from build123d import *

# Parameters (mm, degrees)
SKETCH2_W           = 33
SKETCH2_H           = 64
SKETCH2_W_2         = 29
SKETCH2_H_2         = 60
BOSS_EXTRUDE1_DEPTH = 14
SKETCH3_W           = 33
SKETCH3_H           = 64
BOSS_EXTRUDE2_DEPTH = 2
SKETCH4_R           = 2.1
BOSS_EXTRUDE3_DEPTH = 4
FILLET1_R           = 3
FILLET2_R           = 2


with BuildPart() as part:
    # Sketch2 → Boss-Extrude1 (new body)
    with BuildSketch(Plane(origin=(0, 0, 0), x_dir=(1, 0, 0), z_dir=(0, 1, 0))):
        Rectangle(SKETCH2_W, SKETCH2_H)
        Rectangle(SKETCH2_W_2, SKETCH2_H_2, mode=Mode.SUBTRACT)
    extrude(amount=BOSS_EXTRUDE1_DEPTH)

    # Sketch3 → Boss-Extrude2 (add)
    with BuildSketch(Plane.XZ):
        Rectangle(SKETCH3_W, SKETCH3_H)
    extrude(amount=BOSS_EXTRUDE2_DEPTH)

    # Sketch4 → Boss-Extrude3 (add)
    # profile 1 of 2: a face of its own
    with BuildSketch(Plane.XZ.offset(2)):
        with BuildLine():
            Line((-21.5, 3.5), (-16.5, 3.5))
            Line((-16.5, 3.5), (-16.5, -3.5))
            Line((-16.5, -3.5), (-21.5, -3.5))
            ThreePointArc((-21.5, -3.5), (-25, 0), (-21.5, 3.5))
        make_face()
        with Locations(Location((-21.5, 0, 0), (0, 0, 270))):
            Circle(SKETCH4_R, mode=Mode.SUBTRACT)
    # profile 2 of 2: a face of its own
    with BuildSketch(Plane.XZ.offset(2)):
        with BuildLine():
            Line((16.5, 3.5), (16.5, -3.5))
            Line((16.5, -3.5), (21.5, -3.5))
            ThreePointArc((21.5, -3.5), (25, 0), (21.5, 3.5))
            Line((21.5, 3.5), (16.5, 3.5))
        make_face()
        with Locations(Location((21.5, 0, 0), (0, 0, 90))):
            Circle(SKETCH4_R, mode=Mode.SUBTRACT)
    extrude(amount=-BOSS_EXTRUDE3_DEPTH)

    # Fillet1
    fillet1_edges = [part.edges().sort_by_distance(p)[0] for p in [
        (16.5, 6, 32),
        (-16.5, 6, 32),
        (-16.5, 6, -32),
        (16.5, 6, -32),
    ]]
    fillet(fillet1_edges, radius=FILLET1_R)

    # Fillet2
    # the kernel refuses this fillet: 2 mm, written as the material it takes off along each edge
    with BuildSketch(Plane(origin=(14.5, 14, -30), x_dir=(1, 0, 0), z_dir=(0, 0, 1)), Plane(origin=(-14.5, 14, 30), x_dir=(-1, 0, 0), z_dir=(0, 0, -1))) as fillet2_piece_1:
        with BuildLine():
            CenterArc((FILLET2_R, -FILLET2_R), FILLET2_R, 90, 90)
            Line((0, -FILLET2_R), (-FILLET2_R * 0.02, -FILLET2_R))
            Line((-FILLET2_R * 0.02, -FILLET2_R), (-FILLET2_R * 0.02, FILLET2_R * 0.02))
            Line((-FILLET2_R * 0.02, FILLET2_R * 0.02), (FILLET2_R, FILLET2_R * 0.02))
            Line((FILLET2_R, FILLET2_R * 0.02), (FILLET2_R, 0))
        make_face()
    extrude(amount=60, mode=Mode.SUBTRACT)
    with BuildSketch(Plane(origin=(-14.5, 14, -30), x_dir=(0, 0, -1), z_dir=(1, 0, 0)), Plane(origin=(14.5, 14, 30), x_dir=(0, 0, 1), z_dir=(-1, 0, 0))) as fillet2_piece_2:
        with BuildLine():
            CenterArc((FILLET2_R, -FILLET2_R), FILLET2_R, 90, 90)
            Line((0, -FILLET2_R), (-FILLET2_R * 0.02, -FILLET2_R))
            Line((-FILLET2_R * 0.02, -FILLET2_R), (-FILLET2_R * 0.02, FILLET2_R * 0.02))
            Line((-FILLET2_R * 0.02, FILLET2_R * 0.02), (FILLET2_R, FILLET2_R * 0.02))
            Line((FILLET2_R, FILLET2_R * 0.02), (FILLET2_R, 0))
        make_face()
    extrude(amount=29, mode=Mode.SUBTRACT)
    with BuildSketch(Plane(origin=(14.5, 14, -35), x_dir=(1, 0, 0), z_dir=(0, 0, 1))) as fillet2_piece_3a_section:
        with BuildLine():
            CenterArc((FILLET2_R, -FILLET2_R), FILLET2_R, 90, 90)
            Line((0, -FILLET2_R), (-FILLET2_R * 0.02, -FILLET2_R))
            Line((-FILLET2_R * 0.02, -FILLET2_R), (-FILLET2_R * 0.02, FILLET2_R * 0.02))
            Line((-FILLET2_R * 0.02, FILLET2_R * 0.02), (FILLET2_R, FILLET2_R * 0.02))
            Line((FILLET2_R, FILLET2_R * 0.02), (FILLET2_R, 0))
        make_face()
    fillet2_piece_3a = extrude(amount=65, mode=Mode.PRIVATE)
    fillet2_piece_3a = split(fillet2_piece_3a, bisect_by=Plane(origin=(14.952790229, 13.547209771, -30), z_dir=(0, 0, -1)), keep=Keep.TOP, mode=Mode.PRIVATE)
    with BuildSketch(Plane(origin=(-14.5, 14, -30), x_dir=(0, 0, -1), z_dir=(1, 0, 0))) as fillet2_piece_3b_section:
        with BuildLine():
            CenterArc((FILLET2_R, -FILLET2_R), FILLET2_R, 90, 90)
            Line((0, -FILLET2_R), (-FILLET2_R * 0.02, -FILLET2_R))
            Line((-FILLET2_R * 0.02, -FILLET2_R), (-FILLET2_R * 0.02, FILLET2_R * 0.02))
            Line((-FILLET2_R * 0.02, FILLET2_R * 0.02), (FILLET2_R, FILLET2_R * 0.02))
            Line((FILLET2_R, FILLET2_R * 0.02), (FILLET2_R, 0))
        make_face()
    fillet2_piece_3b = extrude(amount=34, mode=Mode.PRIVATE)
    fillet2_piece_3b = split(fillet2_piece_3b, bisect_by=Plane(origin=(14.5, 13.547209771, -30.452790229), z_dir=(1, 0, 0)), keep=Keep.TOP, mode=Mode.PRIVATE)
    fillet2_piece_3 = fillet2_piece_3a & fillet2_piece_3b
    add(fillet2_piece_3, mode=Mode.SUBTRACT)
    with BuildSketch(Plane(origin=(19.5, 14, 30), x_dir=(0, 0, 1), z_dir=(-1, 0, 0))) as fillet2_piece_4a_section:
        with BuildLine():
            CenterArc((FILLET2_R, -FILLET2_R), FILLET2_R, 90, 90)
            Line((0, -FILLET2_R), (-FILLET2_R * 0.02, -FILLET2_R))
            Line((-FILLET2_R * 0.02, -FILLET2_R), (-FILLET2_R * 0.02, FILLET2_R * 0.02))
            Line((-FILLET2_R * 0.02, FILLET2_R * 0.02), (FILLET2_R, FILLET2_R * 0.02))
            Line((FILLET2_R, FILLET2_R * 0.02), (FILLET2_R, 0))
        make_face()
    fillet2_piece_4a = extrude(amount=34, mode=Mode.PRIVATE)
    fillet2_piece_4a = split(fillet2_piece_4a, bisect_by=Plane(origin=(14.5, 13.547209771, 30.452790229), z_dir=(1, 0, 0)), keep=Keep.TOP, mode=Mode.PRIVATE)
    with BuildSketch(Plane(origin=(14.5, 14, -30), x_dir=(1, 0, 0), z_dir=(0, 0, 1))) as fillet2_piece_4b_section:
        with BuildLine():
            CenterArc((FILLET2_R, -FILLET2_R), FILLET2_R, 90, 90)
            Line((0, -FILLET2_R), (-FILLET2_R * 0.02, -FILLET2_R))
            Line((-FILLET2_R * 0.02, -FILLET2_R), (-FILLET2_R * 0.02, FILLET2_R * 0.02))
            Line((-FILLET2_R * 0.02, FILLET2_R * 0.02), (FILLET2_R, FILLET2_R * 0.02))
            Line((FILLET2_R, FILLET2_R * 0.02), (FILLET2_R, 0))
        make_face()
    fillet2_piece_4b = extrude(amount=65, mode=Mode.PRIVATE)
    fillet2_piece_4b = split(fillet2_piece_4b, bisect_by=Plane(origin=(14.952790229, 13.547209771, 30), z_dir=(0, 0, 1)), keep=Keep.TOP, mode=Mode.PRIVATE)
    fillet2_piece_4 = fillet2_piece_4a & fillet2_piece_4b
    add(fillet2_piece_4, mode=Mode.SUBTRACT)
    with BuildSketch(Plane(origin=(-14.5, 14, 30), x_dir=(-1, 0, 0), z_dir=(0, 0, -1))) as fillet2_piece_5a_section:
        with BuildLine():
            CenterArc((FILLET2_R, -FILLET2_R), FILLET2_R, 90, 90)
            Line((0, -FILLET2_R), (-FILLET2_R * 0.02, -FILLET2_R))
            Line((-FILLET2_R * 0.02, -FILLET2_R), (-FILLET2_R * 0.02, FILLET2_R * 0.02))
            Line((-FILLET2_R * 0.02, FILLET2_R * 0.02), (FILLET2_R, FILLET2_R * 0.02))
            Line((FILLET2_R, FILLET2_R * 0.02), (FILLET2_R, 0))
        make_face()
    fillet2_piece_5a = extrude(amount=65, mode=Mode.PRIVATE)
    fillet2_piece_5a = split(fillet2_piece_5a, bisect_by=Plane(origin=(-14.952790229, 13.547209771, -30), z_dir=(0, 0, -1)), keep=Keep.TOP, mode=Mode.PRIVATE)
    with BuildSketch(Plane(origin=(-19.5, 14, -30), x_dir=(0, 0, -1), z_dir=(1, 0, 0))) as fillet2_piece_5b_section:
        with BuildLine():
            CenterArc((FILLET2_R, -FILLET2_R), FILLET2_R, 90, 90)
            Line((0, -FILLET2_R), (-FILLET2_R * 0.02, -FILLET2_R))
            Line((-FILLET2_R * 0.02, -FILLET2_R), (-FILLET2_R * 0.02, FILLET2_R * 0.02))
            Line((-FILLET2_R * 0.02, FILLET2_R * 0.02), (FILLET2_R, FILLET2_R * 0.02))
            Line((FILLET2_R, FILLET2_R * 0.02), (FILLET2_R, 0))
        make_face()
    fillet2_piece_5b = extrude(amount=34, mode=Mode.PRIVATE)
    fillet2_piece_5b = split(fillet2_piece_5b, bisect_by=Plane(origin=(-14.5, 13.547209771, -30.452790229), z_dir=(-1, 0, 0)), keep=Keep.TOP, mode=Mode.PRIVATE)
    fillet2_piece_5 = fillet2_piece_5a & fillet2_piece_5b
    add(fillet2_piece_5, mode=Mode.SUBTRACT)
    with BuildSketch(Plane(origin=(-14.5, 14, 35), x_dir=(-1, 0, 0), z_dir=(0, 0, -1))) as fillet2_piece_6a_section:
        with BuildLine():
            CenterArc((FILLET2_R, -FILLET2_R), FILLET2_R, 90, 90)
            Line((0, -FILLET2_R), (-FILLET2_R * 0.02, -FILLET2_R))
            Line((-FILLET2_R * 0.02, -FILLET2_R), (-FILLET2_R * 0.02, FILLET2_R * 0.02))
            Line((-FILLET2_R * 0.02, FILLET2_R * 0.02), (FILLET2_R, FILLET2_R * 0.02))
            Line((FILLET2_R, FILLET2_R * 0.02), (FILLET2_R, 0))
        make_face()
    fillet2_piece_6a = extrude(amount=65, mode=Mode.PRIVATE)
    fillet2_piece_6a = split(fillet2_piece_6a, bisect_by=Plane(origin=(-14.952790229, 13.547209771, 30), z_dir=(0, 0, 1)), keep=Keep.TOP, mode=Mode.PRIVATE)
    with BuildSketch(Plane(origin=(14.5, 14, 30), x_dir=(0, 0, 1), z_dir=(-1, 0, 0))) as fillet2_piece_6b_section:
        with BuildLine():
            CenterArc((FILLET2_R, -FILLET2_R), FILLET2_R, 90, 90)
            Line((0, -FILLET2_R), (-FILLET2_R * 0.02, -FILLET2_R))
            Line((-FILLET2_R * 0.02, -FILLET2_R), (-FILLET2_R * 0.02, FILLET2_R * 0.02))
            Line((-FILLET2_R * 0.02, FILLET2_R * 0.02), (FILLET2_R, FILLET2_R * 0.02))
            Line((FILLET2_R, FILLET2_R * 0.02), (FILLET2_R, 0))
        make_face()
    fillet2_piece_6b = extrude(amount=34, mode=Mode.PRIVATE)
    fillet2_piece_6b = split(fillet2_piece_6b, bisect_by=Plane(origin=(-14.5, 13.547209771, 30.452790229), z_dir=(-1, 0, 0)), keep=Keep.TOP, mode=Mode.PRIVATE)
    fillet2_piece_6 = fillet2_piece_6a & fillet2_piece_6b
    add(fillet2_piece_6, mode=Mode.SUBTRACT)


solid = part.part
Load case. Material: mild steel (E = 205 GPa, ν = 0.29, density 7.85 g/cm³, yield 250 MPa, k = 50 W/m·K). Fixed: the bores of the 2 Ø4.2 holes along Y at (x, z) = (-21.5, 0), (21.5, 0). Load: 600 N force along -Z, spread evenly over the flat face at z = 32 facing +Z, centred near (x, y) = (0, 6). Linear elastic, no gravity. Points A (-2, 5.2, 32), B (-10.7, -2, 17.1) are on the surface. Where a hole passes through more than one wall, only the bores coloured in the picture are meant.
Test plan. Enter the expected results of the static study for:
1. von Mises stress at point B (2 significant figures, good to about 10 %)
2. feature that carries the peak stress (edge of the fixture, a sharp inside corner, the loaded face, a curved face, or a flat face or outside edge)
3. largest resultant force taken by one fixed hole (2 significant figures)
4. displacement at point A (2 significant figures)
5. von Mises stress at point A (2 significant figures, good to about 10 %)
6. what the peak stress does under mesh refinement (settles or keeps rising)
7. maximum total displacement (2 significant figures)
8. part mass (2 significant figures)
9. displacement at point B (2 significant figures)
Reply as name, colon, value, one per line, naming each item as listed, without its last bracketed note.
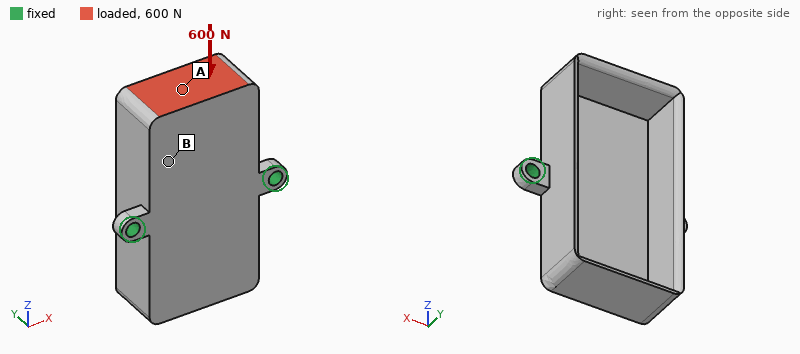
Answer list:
von Mises stress at point B: 12 MPa
feature that carries the peak stress: edge of the fixture
largest resultant force taken by one fixed hole: 300 N
displacement at point A: 42 µm
von Mises stress at point A: 33 MPa
what the peak stress does under mesh refinement: keeps rising
maximum total displacement: 62 µm
part mass: 74 g
displacement at point B: 17 µm
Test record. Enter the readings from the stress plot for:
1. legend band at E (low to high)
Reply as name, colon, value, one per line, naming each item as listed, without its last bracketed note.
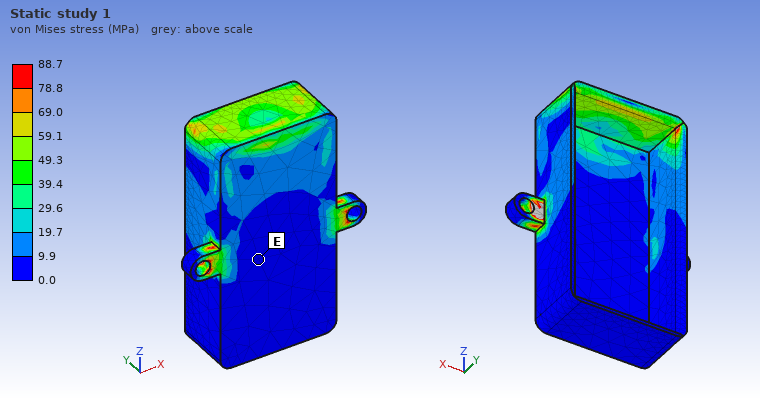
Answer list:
legend band at E: 0.0 to 9.9 MPa
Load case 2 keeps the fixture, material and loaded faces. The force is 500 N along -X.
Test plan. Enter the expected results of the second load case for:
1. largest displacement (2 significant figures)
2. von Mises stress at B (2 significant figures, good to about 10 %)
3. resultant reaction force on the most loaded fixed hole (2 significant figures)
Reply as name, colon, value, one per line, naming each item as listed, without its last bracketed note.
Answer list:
largest displacement: 52 µm
von Mises stress at B: 15 MPa
resultant reaction force on the most loaded fixed hole: 500 N
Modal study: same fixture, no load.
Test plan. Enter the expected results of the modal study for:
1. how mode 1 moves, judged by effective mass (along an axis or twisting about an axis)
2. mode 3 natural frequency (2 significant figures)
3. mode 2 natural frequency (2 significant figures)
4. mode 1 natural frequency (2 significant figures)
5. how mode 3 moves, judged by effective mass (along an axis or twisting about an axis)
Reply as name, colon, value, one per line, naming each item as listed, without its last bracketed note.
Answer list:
how mode 1 moves, judged by effective mass: twisting about X
mode 3 natural frequency: 5700 Hz
mode 2 natural frequency: 3000 Hz
mode 1 natural frequency: 1600 Hz
how mode 3 moves, judged by effective mass: along Y
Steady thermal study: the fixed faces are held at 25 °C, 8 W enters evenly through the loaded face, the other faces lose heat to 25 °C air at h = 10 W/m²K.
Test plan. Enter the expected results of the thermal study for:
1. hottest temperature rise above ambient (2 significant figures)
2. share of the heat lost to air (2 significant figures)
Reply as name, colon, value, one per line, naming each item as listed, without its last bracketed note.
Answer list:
hottest temperature rise above ambient: 61 K
share of the heat lost to air: 24 %
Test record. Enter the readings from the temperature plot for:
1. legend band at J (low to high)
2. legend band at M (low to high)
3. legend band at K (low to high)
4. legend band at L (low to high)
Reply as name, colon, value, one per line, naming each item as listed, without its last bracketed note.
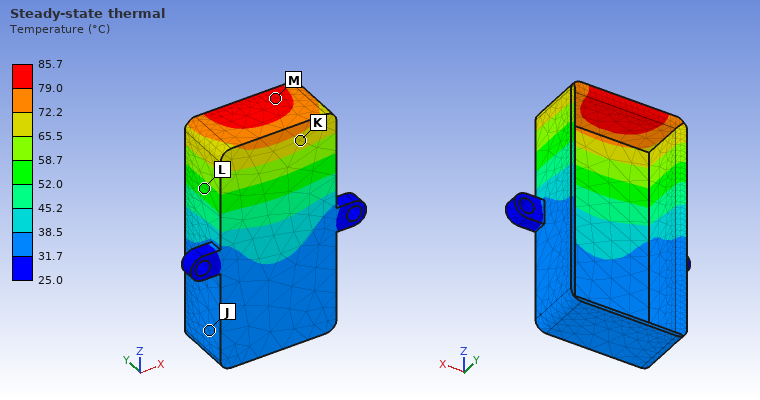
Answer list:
legend band at J: 31.7 to 38.5 °C
legend band at M: 79.0 to 85.7 °C
legend band at K: 65.5 to 72.2 °C
legend band at L: 52.0 to 58.7 °C
